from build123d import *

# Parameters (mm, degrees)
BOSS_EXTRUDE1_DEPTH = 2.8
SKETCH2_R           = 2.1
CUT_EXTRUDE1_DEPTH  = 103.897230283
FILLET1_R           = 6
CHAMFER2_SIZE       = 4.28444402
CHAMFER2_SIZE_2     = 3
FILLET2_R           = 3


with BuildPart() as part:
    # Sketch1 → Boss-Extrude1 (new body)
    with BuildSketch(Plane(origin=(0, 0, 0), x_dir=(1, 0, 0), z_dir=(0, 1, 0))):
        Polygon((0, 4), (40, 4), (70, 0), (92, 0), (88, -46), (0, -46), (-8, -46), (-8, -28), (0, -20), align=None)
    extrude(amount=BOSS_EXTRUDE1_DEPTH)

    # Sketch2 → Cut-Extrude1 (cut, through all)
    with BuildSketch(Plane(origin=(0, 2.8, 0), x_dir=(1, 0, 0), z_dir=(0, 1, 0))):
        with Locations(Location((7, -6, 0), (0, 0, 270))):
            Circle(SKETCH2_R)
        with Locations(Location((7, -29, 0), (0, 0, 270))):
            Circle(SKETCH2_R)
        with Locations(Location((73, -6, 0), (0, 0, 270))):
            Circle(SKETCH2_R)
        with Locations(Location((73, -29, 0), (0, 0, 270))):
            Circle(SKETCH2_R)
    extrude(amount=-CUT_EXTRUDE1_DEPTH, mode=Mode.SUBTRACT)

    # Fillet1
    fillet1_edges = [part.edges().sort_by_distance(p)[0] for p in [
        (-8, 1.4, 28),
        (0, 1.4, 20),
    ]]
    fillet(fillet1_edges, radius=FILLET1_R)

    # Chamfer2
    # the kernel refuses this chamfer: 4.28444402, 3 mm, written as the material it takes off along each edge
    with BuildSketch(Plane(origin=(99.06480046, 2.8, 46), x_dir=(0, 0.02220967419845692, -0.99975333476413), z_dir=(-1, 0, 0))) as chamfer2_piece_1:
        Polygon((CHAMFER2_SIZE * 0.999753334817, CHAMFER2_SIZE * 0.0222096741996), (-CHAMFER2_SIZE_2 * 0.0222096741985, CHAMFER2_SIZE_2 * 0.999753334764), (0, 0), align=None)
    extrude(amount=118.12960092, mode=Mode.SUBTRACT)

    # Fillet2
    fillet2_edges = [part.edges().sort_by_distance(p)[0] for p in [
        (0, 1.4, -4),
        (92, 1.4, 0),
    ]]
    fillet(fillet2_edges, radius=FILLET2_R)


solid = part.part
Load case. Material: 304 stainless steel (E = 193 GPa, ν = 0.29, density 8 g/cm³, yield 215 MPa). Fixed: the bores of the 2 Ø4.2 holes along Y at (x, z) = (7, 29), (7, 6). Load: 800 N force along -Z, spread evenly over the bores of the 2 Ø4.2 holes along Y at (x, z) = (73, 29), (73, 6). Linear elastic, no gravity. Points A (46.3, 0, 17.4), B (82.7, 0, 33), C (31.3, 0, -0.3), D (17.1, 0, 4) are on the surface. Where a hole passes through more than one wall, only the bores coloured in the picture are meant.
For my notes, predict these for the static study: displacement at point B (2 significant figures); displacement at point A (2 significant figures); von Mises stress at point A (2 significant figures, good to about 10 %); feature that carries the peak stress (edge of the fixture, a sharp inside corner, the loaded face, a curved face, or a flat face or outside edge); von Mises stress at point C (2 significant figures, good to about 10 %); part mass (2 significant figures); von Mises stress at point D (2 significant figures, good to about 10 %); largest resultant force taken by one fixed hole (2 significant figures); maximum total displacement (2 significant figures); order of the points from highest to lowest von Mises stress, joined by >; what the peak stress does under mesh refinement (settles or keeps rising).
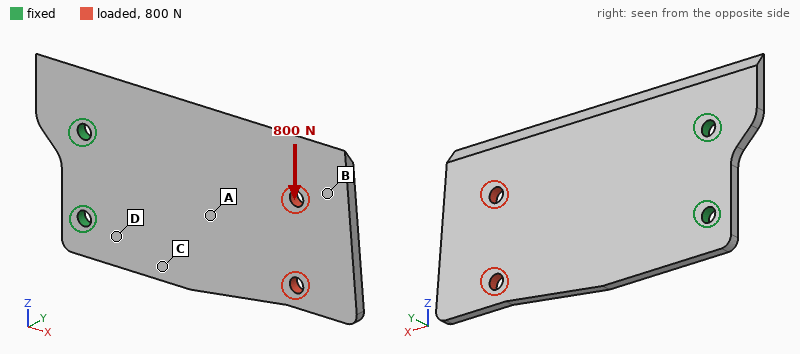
39 µm
16 µm
16 MPa
edge of the fixture
28 MPa
95 g
40 MPa
2.1 kN
44 µm
D > C > A > B
keeps rising
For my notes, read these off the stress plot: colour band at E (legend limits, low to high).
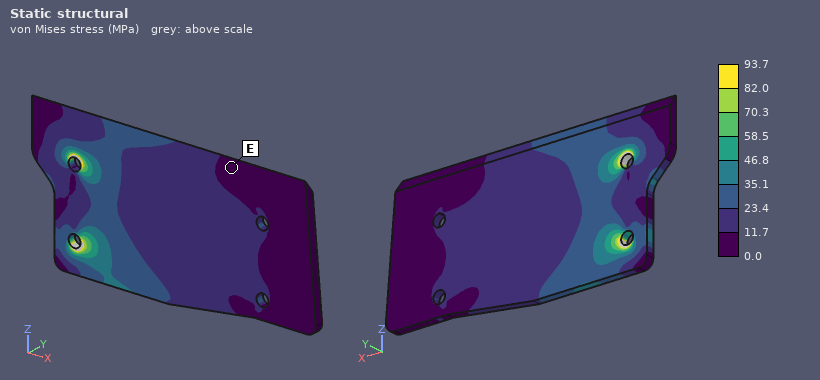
0.0 to 11.7 MPa
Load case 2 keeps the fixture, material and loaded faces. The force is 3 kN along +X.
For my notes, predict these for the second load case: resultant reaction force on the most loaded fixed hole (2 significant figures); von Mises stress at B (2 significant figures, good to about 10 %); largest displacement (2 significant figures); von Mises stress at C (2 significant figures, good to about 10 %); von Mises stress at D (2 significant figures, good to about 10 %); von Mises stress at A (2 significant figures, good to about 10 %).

1.5 kN
7.4 MPa
13 µm
26 MPa
32 MPa
25 MPa
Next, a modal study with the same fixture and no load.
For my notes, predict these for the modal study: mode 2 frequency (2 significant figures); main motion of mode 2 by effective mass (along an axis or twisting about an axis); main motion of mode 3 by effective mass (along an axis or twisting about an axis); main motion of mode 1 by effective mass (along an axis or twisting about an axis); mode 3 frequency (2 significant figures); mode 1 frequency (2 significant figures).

1300 Hz
twisting about X
along Y
along Y
2000 Hz
340 Hz
